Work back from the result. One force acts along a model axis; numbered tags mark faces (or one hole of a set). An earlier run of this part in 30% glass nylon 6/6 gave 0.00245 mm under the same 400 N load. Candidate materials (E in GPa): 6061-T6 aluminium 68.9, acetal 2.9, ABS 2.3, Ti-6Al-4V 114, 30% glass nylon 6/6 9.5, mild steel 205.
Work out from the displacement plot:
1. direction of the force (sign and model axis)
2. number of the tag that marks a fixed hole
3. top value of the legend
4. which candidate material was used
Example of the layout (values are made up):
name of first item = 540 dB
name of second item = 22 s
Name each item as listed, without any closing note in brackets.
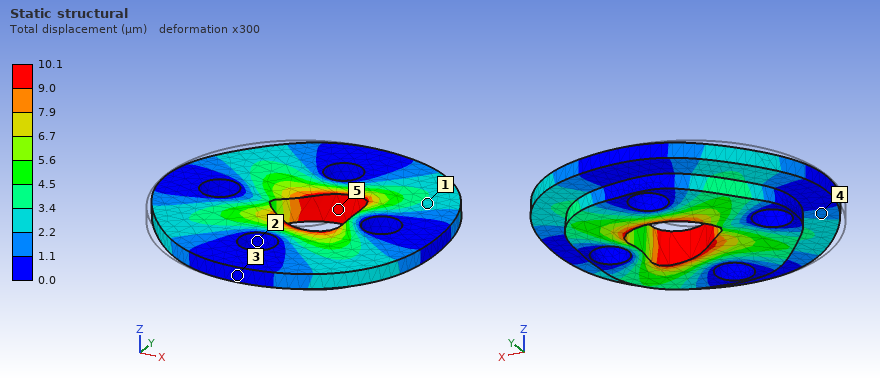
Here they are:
direction of the force = +X
number of the tag that marks a fixed hole = 2
top value of the legend = 10.1 µm
which candidate material was used = ABS
